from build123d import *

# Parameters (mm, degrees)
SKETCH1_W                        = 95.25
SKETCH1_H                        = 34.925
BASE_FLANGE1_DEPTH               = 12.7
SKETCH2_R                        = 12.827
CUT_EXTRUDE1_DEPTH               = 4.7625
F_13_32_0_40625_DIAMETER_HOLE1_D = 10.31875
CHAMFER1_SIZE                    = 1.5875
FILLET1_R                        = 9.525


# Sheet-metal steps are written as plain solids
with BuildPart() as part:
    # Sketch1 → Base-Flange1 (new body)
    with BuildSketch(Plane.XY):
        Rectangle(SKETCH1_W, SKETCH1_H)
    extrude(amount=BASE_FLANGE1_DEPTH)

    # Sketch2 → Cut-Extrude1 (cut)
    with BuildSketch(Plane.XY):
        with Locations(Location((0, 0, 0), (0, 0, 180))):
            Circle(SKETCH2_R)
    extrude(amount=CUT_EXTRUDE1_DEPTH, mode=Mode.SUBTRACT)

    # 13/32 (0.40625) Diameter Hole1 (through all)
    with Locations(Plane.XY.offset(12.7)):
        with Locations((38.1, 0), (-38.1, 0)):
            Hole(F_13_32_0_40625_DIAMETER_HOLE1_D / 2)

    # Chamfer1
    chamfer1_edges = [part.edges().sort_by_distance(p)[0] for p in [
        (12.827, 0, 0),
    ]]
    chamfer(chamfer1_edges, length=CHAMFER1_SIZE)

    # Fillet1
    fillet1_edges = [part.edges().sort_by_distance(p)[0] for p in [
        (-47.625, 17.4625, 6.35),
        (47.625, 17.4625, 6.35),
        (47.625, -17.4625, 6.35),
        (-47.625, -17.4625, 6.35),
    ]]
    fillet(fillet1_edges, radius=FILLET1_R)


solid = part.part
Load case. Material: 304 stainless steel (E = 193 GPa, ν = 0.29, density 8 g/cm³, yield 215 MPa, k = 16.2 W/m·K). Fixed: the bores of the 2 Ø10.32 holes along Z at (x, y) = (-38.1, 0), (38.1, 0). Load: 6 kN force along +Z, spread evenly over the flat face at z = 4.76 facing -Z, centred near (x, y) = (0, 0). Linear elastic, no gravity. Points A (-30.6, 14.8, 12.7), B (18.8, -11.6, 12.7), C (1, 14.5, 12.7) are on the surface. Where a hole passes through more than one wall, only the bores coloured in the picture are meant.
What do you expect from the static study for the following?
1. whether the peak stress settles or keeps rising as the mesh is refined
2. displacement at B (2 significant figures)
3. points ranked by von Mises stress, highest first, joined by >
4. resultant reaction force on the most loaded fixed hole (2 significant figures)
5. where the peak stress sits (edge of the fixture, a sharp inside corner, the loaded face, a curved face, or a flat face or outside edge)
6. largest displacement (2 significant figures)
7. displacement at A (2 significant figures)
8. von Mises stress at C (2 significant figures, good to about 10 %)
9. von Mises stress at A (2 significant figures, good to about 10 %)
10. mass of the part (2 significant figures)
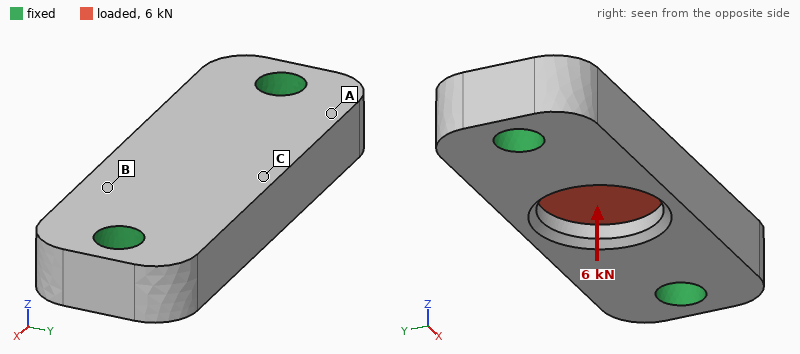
keeps rising
8.6 µm
C > A > B
3.3 kN
edge of the fixture
18 µm
2.9 µm
55 MPa
24 MPa
290 g
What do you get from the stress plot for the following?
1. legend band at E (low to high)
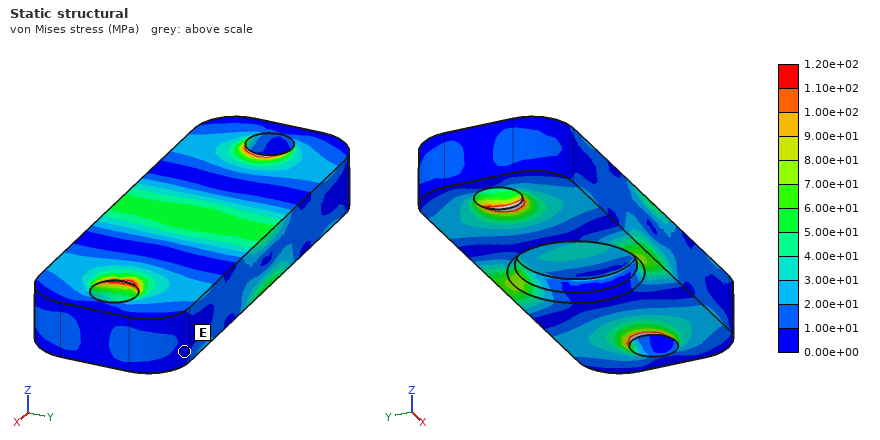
0.00e+00 to 1.00e+01 MPa
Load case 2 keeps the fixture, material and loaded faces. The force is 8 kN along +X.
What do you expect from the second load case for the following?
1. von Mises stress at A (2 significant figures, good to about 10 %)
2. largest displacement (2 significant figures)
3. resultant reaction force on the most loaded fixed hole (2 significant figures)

5.8 MPa
3.4 µm
4.0 kN
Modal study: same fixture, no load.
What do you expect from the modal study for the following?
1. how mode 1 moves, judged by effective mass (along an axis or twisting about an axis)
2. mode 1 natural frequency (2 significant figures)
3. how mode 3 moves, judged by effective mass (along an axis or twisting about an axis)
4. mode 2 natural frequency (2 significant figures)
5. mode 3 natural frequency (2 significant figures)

along Z
9900 Hz
along Y
13 kHz
15 kHz
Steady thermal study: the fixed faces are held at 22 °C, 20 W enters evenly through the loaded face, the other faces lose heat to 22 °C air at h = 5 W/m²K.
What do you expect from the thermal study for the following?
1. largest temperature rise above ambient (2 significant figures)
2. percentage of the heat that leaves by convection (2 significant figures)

58 K
4.3 %
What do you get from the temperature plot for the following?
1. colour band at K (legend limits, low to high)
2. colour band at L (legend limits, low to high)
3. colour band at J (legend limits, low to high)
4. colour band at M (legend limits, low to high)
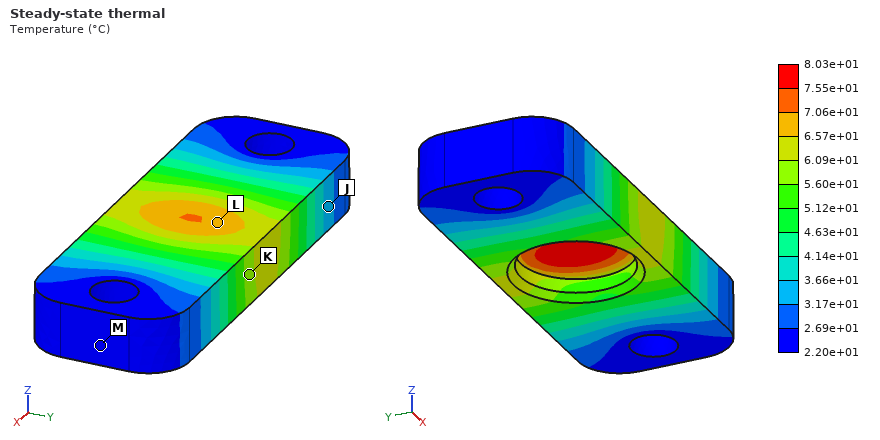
5.60e+01 to 6.09e+01 °C
6.57e+01 to 7.06e+01 °C
3.17e+01 to 3.66e+01 °C
2.20e+01 to 2.69e+01 °C
